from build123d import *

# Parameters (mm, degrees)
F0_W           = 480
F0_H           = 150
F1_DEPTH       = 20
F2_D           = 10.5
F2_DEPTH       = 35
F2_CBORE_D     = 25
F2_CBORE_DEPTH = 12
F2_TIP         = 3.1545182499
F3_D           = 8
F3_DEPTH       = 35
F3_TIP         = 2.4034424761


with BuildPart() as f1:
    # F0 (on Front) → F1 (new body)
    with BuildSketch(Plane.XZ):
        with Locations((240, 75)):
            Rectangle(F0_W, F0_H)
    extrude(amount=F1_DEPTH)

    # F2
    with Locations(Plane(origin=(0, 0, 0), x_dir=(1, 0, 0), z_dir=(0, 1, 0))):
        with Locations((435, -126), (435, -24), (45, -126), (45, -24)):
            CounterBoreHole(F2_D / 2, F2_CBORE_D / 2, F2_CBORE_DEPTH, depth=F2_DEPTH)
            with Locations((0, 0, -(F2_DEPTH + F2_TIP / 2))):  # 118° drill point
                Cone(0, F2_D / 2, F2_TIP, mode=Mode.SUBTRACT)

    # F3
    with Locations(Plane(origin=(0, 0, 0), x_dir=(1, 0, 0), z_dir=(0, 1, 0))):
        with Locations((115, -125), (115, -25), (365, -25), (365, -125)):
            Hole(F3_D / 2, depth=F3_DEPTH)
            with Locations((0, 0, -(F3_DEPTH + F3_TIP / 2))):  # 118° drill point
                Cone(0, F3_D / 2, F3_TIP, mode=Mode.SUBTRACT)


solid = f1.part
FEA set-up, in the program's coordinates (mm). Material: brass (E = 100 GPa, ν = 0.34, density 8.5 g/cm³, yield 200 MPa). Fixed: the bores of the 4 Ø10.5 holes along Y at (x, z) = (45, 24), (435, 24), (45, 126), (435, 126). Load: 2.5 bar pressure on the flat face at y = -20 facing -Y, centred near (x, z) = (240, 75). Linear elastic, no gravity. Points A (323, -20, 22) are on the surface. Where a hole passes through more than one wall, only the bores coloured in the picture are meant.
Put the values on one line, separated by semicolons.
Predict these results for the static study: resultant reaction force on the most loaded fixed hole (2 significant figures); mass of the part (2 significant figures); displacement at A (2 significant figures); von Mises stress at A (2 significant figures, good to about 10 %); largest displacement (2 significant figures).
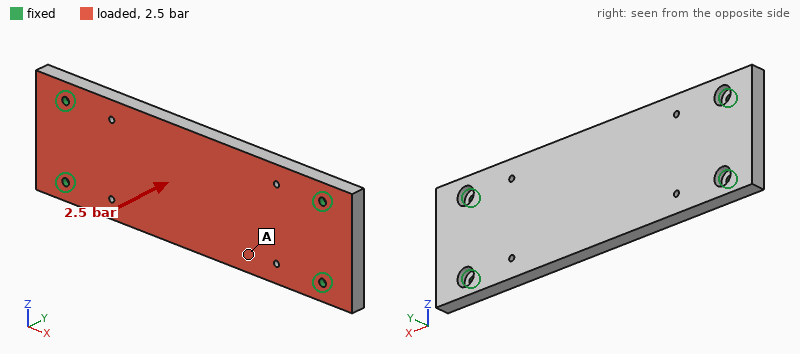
9.3 kN; 12 kg; 0.31 mm; 16 MPa; 0.43 mm
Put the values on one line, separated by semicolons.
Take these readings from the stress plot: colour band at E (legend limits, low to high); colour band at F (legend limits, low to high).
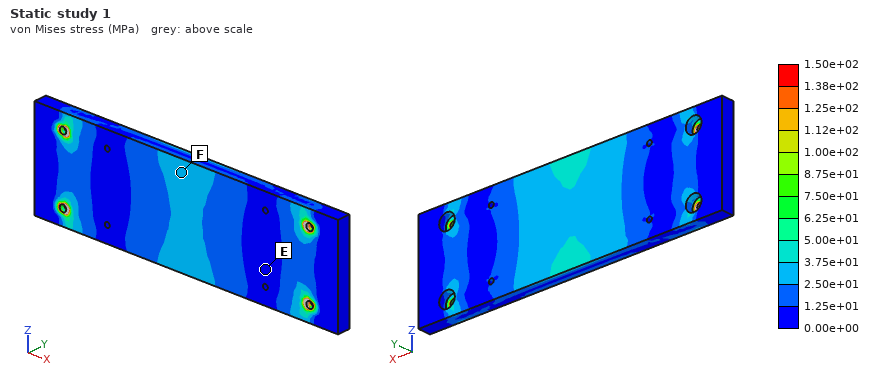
0.00e+00 to 1.25e+01 MPa; 2.50e+01 to 3.75e+01 MPa
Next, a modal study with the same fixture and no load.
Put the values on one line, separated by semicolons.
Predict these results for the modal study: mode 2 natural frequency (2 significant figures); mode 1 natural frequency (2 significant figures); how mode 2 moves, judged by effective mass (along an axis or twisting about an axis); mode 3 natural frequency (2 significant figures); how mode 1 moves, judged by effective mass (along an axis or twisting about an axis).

770 Hz; 330 Hz; twisting about X; 920 Hz; along Y
